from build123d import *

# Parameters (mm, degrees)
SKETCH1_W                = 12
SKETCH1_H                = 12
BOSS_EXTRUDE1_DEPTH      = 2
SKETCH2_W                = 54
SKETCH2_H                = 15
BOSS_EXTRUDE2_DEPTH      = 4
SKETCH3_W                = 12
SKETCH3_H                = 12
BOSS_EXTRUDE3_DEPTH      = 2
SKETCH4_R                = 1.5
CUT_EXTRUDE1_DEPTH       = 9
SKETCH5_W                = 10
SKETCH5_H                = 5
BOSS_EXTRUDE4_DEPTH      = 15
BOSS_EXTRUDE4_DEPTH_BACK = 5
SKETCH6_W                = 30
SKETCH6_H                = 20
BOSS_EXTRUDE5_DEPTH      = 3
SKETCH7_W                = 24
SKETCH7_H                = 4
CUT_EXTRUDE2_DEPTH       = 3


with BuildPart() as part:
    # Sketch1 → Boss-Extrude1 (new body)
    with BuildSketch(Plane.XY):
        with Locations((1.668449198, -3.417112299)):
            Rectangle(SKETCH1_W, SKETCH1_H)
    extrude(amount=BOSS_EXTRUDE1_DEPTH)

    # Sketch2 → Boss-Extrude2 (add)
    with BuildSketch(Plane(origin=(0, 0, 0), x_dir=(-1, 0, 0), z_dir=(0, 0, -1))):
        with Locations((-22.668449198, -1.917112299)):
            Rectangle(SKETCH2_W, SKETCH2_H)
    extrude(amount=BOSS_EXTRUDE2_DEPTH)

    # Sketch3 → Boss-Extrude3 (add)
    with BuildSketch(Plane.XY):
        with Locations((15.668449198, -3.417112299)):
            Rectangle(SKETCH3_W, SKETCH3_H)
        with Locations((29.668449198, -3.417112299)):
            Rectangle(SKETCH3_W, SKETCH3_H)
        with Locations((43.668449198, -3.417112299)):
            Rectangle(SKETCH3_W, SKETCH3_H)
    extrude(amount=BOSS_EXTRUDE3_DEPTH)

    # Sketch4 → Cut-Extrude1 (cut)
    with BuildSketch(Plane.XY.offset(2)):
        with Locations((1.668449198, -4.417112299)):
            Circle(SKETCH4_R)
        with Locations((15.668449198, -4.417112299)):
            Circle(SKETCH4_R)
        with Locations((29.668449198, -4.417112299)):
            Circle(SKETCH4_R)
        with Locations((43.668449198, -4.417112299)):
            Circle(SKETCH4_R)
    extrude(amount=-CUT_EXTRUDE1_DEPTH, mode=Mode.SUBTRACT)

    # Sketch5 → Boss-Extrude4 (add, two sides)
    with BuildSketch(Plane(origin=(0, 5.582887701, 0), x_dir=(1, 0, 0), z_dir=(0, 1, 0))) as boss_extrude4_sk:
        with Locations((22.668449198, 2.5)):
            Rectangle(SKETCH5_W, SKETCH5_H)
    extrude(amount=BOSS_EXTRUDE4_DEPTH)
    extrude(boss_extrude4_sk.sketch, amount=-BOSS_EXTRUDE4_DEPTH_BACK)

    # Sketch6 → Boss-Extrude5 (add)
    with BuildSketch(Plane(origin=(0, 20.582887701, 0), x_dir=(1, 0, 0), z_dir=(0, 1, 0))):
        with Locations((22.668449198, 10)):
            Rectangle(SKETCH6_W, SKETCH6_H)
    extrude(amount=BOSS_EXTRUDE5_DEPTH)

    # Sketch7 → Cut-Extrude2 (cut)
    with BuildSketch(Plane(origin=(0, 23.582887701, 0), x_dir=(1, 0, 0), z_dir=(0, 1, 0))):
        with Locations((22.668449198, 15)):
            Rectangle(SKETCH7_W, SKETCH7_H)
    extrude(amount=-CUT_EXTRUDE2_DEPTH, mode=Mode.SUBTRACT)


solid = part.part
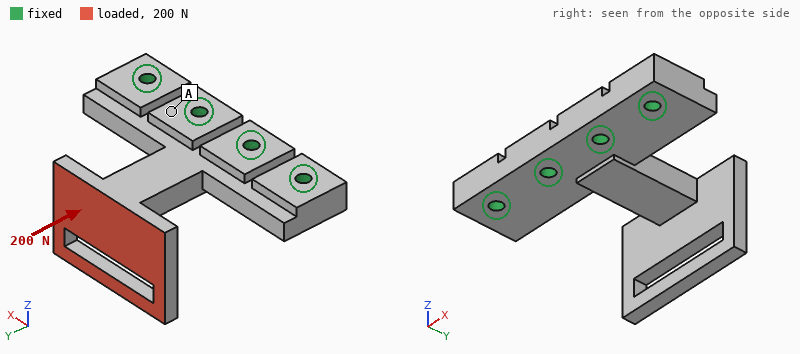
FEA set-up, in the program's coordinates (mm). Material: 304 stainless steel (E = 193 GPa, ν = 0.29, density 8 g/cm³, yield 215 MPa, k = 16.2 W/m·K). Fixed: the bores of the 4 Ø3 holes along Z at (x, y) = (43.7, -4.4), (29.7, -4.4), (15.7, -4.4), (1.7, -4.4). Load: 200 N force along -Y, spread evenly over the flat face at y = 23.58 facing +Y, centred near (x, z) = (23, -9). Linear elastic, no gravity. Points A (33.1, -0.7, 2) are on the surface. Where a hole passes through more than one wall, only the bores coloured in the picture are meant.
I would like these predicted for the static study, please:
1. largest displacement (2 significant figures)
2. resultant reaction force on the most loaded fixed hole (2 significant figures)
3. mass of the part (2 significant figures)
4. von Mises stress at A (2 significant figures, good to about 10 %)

47 µm
110 N
52 g
4.5 MPa
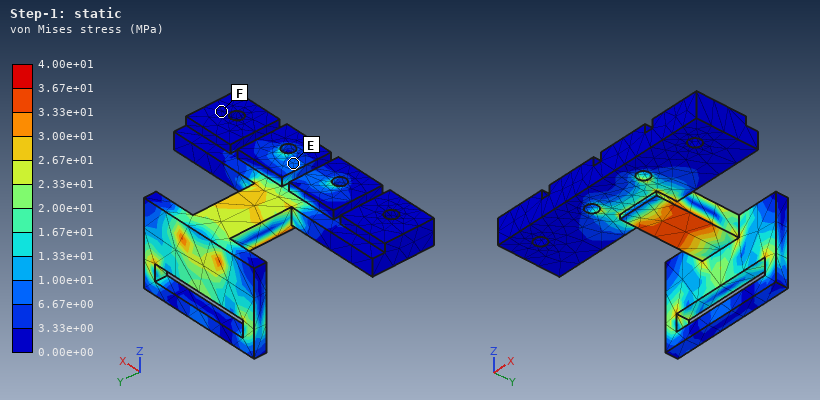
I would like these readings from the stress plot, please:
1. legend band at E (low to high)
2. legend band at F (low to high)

6.67e+00 to 1.00e+01 MPa
0.00e+00 to 3.33e+00 MPa
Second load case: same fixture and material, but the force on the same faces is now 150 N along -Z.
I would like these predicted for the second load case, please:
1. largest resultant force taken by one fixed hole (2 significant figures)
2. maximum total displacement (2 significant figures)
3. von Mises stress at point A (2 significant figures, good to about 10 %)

82 N
56 µm
12 MPa
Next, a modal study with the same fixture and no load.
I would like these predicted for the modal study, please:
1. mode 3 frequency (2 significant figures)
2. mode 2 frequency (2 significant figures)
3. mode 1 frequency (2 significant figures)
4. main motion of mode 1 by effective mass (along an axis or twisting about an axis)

5900 Hz
3700 Hz
2600 Hz
along Z
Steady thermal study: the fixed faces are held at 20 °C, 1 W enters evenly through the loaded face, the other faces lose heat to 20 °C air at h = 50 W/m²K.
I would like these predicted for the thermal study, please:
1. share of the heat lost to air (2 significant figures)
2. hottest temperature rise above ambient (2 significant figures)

70 %
13 K
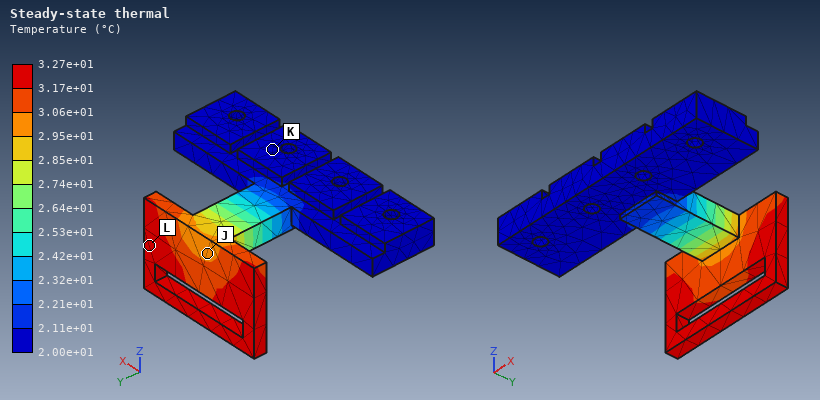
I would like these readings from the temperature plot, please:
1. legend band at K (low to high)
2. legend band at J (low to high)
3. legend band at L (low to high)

2.00e+01 to 2.11e+01 °C
2.95e+01 to 3.06e+01 °C
3.17e+01 to 3.27e+01 °C
